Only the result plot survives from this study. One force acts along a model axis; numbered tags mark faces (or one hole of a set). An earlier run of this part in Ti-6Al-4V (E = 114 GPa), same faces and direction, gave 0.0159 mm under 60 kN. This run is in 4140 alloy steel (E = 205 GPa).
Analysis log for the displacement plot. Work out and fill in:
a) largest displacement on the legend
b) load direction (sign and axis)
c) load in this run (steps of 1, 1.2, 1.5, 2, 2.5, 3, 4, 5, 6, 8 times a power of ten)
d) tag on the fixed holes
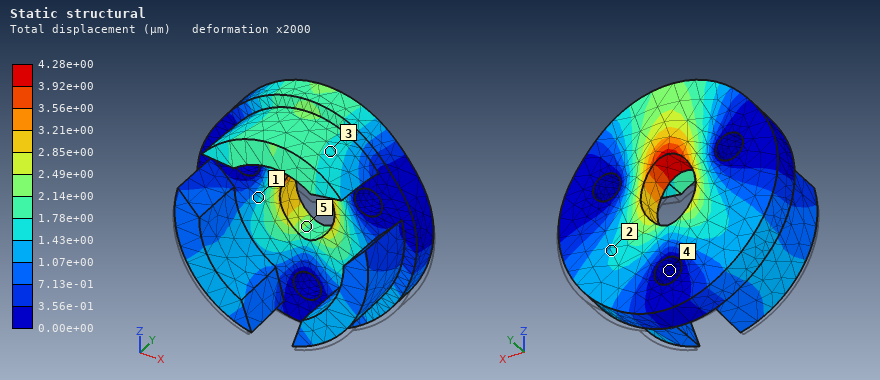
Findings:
4.28e+00 µm
+Z
30 kN
4
